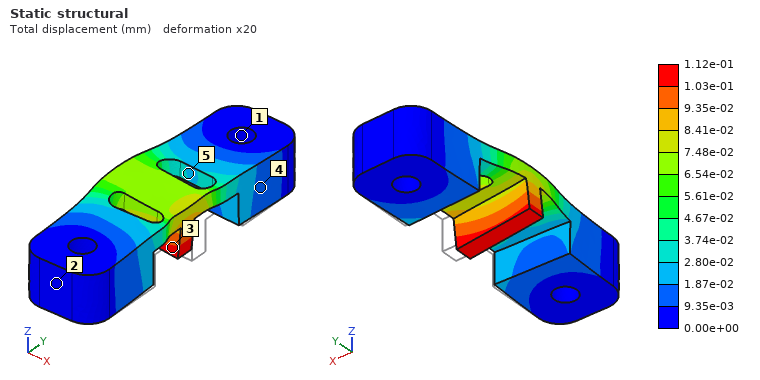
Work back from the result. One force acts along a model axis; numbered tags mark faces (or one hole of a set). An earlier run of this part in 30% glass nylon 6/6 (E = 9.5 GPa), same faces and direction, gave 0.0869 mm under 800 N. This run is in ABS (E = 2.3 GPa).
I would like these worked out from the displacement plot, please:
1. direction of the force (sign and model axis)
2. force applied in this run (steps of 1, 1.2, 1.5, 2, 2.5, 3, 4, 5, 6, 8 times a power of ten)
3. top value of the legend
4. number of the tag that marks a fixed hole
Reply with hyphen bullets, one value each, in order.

- -X
- 250 N
- 1.12e-01 mm
- 1
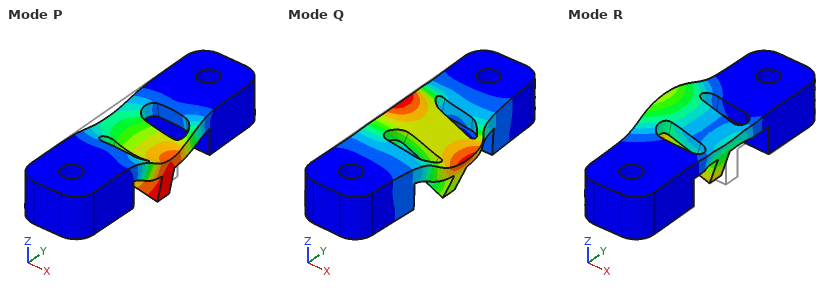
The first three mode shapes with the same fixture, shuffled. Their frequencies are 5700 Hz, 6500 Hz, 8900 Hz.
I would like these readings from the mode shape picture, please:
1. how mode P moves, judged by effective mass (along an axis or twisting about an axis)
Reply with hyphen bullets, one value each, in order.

- along Z
